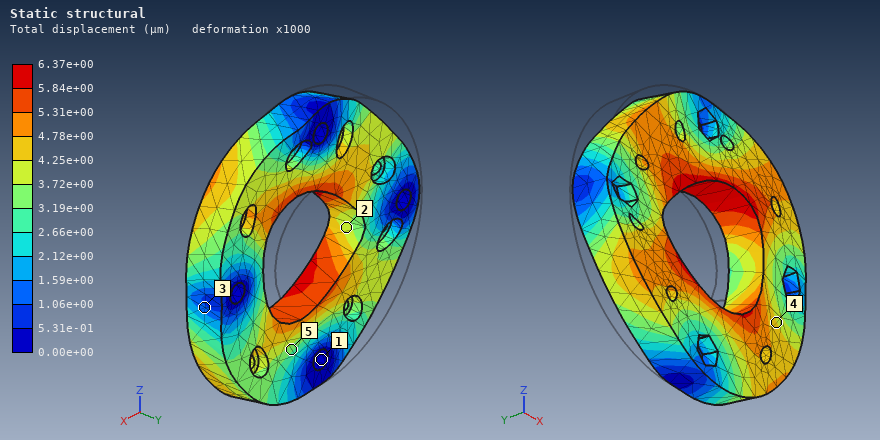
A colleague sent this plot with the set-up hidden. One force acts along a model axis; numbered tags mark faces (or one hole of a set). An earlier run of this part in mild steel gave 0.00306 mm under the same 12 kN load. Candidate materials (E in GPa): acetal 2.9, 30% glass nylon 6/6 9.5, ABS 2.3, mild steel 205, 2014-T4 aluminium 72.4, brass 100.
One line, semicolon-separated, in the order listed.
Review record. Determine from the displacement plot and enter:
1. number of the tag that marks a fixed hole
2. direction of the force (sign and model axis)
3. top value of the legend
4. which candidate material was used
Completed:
1; +X; 6.37e+00 µm; brass
